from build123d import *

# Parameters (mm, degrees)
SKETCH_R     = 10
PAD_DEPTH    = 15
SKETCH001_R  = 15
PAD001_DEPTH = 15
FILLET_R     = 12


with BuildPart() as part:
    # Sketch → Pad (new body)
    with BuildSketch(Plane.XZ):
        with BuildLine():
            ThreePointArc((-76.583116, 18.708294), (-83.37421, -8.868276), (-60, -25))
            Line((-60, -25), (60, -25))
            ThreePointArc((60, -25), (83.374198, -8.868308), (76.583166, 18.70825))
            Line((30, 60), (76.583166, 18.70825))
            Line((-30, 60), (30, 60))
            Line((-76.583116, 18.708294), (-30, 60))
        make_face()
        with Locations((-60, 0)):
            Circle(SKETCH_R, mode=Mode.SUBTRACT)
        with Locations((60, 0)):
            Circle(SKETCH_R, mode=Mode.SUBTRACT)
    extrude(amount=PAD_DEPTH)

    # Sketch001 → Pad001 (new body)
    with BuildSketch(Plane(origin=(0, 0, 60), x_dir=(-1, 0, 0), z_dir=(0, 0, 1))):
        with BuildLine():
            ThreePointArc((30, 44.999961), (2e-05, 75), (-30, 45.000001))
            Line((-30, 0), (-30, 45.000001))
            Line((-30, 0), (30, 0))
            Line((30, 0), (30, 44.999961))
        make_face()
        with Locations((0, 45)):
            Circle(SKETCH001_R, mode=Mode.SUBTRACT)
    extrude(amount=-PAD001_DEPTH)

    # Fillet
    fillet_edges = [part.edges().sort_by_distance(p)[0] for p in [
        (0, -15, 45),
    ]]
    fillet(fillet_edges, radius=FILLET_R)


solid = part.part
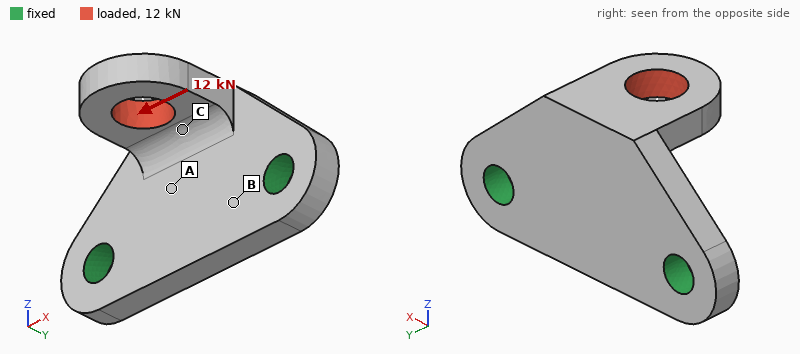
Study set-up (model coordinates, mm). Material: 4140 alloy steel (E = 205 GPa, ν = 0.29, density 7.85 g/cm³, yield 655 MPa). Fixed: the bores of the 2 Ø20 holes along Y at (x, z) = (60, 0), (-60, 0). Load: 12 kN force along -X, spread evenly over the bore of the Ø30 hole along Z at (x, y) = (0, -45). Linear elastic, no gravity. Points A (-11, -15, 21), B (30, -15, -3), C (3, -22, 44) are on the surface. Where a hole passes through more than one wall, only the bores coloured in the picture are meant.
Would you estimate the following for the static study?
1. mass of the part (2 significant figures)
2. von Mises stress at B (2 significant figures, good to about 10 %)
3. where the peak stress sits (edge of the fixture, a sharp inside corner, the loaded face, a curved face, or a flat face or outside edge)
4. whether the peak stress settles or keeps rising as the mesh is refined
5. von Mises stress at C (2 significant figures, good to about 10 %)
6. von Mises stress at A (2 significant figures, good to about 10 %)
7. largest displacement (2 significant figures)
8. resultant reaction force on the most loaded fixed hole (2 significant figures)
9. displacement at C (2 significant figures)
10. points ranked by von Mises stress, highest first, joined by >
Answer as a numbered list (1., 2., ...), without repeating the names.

1. 1.6 kg
2. 16 MPa
3. a sharp inside corner
4. keeps rising
5. 88 MPa
6. 45 MPa
7. 96 µm
8. 9.1 kN
9. 19 µm
10. C > A > B
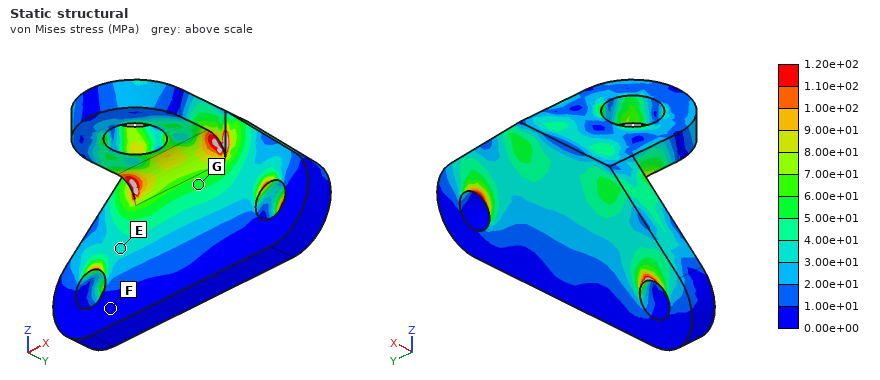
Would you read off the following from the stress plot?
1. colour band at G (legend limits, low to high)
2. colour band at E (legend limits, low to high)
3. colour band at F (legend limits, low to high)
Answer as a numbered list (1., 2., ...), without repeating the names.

1. 5.00e+01 to 6.00e+01 MPa
2. 3.00e+01 to 4.00e+01 MPa
3. 0.00e+00 to 1.00e+01 MPa
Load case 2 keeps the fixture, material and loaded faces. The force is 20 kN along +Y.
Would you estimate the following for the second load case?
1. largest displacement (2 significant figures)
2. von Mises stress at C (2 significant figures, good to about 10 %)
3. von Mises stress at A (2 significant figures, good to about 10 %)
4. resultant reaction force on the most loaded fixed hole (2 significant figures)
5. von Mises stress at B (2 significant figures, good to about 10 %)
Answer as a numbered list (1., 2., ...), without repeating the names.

1. 0.38 mm
2. 35 MPa
3. 98 MPa
4. 10 kN
5. 94 MPa
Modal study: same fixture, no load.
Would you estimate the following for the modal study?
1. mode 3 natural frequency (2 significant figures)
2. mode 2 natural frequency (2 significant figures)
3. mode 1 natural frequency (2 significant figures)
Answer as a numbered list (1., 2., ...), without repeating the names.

1. 3700 Hz
2. 3700 Hz
3. 1800 Hz
